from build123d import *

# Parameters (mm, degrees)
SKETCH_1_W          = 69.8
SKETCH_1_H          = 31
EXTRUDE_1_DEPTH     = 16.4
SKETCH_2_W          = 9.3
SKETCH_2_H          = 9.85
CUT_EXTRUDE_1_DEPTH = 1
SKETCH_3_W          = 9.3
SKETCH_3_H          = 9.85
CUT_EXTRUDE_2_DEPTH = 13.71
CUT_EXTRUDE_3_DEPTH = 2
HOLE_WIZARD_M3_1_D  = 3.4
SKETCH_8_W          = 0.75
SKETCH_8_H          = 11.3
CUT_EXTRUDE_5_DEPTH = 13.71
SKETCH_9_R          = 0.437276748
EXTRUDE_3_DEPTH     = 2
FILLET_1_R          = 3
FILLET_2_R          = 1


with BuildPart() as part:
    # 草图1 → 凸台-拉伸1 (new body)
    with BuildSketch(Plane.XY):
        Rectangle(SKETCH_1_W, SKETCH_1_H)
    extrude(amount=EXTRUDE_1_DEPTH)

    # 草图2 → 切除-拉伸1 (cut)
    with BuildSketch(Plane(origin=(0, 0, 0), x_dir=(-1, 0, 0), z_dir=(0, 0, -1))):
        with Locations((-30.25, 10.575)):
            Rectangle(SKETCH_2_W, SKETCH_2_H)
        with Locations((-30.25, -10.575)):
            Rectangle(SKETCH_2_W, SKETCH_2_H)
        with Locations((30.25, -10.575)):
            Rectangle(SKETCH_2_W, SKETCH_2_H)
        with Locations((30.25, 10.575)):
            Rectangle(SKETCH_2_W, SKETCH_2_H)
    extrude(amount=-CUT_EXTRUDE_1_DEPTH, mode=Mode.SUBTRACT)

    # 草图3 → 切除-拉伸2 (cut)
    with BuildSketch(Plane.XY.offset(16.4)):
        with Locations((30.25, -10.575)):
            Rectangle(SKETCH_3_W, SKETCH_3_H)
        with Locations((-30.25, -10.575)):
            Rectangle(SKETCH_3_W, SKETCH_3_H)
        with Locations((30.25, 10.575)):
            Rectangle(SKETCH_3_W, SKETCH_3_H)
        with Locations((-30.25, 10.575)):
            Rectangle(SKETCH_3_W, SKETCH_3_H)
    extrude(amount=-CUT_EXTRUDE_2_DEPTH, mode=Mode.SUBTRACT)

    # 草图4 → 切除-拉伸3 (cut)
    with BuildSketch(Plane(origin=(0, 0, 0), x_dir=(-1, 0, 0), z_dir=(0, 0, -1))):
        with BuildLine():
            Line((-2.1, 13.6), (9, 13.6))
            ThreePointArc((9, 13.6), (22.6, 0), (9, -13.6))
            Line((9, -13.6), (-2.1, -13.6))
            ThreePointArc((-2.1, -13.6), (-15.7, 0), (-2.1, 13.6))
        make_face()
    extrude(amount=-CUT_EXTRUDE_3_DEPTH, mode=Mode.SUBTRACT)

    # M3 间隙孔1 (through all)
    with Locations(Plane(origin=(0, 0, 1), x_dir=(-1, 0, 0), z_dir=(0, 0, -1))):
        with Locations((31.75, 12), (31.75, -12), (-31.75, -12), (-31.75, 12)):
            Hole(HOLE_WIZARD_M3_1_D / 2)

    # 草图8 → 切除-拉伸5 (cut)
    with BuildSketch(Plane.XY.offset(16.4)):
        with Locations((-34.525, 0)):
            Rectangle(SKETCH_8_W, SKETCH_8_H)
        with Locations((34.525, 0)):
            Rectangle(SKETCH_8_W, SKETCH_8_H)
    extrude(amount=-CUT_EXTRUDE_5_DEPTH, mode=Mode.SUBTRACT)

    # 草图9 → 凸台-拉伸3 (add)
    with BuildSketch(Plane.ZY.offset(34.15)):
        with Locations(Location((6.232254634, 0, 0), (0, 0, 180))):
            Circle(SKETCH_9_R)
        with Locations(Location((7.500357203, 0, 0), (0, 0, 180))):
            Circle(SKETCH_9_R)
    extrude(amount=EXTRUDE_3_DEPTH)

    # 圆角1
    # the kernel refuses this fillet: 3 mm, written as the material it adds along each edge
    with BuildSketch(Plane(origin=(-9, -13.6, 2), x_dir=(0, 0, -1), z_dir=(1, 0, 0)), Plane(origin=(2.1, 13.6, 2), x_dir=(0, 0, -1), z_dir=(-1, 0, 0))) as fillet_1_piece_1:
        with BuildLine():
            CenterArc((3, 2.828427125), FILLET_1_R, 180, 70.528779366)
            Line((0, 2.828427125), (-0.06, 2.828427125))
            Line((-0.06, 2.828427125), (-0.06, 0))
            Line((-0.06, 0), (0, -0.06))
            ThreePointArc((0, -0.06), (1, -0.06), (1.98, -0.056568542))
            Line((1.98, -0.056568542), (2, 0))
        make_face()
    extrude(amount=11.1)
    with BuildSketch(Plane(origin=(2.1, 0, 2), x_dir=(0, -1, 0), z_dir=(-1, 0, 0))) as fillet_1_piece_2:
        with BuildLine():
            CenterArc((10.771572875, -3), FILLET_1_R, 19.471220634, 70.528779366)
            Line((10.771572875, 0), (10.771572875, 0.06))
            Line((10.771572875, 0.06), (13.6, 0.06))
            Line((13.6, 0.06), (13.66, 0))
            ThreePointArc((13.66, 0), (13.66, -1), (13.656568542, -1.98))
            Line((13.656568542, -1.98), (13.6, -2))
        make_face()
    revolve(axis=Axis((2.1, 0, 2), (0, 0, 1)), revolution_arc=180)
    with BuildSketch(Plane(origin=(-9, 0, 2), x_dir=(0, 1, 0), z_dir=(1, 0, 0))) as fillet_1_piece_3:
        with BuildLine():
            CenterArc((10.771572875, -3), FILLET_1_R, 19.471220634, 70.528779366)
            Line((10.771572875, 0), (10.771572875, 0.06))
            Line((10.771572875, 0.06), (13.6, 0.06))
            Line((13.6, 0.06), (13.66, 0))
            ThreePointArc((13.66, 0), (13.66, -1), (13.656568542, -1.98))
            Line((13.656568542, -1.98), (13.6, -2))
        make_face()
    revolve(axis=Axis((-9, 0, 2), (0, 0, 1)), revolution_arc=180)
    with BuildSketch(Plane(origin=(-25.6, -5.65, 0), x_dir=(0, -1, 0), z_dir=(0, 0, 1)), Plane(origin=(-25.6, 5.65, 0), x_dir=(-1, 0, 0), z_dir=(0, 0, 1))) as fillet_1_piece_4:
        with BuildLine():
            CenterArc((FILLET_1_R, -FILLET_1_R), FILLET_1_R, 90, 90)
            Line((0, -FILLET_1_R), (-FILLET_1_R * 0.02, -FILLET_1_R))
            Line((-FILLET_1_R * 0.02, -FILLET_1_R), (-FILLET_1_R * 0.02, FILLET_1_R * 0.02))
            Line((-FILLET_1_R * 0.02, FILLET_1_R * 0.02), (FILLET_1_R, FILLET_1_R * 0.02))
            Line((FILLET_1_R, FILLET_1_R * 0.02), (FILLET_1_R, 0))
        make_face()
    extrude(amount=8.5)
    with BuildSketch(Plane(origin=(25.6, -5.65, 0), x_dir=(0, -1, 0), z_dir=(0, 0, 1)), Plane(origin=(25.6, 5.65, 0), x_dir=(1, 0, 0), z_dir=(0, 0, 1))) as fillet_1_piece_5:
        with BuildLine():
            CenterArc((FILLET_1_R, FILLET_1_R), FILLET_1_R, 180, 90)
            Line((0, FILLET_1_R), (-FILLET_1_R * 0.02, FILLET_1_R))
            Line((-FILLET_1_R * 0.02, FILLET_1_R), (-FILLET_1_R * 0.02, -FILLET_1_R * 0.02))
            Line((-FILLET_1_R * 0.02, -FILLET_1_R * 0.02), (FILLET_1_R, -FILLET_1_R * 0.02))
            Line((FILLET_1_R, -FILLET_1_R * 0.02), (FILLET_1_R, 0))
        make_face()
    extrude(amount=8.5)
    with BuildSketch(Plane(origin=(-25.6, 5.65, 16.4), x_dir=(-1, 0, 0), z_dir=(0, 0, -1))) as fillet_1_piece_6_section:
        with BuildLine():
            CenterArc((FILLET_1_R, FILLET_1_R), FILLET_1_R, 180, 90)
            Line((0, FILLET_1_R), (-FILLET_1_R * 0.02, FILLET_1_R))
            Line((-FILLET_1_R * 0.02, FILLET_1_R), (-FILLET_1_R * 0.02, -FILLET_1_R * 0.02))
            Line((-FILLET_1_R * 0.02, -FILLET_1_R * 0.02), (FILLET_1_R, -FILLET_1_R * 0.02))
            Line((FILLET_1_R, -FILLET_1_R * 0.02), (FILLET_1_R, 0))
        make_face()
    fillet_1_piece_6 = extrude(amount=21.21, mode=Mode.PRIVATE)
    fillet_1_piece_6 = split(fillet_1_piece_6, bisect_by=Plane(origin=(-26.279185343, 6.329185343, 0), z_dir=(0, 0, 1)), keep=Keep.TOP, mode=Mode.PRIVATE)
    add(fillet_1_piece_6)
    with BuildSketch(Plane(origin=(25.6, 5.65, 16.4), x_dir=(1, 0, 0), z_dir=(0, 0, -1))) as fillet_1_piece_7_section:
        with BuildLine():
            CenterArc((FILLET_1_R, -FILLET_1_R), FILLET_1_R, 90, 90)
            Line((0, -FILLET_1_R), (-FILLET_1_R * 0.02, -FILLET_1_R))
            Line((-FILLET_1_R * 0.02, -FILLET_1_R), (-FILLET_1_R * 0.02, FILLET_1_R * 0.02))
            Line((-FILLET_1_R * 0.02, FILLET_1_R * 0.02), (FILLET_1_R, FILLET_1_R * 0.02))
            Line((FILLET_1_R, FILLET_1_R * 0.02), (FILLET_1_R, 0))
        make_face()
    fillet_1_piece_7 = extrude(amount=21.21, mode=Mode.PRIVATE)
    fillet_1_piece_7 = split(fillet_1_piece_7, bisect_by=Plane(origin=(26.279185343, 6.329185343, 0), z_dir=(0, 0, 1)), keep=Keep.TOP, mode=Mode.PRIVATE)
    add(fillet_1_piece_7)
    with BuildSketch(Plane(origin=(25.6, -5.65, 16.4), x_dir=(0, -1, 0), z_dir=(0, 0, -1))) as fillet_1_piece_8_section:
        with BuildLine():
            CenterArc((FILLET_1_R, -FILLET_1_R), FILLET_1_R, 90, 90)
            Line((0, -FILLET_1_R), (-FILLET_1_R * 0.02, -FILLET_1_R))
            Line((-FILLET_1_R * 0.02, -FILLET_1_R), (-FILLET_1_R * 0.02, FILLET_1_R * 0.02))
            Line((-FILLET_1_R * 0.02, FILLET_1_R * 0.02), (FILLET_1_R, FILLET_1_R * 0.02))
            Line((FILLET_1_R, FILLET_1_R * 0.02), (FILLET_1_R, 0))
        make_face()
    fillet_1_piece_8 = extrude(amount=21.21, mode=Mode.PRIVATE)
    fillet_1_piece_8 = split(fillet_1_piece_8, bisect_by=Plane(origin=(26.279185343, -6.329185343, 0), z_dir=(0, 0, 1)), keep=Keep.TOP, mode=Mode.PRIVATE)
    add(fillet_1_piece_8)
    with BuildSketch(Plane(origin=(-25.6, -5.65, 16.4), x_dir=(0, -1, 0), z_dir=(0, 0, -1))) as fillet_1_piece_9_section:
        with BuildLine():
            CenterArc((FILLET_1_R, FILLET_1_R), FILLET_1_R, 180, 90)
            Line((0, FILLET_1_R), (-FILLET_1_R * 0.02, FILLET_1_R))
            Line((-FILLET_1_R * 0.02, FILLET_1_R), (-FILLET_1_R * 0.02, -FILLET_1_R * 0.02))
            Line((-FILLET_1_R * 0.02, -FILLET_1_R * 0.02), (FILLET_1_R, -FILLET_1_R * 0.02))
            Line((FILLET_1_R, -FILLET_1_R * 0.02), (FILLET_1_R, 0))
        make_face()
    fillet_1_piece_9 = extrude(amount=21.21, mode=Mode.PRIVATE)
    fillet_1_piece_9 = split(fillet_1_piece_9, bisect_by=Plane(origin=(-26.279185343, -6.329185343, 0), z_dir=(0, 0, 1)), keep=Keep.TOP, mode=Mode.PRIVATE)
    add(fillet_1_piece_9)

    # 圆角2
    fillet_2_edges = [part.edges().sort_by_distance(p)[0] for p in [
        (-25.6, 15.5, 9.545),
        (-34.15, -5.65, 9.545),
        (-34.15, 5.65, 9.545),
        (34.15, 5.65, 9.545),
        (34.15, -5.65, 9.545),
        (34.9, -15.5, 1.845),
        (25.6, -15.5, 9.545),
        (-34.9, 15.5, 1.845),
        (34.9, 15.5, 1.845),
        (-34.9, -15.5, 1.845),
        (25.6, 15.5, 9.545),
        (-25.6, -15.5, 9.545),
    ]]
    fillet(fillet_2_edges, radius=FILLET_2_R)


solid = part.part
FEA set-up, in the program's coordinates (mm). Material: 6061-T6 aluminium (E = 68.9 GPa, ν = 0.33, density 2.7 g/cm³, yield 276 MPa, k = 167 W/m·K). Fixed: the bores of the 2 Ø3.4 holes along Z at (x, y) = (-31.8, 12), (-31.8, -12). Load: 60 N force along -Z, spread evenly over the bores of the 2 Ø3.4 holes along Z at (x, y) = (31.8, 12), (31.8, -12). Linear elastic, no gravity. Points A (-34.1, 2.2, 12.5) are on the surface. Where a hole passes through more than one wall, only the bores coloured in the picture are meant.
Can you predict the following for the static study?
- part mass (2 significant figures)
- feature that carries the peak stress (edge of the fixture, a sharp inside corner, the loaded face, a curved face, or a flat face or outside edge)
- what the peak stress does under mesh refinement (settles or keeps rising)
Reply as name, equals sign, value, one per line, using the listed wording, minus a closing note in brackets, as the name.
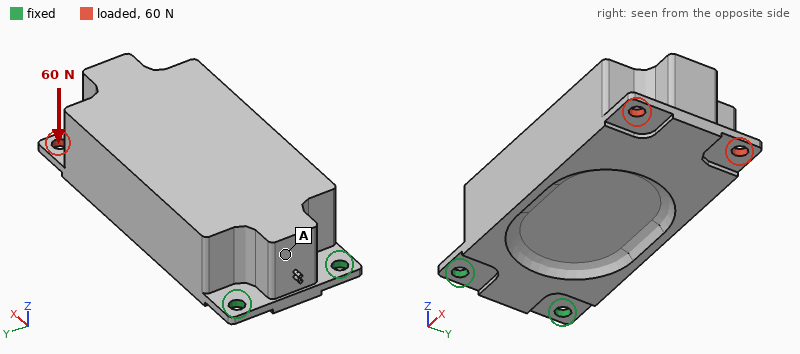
part mass = 76 g
feature that carries the peak stress = edge of the fixture
what the peak stress does under mesh refinement = keeps rising
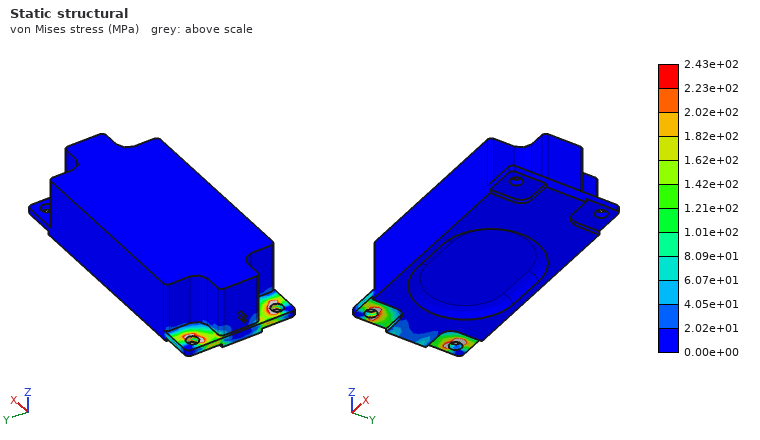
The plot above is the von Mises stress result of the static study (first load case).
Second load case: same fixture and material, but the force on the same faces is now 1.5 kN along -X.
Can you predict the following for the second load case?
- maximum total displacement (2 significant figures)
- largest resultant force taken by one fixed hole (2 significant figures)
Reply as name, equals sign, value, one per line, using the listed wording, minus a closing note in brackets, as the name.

maximum total displacement = 36 µm
largest resultant force taken by one fixed hole = 760 N
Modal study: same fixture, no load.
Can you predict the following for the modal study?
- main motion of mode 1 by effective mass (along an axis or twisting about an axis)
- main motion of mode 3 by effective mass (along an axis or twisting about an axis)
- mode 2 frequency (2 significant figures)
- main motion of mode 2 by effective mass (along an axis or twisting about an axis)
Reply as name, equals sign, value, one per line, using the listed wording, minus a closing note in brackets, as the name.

main motion of mode 1 by effective mass = along Z
main motion of mode 3 by effective mass = twisting about X
mode 2 frequency = 2500 Hz
main motion of mode 2 by effective mass = along Y
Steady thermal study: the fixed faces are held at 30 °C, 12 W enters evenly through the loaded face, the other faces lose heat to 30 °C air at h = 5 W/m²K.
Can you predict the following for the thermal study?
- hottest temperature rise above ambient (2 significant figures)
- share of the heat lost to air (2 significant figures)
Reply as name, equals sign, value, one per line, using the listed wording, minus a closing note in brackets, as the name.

hottest temperature rise above ambient = 36 K
share of the heat lost to air = 4.5 %
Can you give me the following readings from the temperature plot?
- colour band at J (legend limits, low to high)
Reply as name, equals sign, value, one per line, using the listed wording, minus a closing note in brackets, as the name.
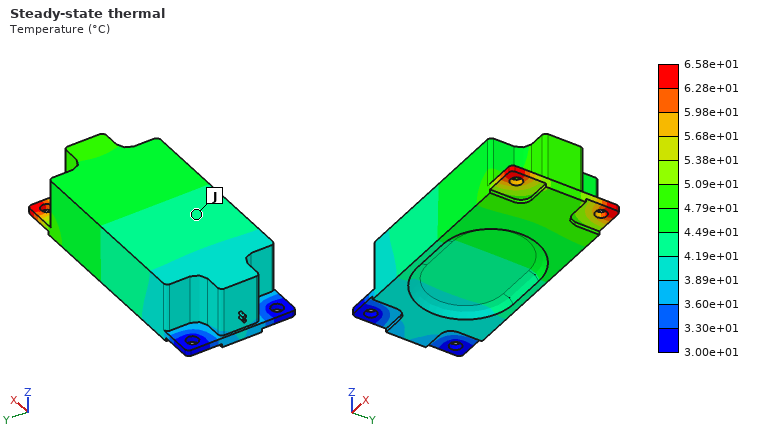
colour band at J = 4.19e+01 to 4.49e+01 °C
